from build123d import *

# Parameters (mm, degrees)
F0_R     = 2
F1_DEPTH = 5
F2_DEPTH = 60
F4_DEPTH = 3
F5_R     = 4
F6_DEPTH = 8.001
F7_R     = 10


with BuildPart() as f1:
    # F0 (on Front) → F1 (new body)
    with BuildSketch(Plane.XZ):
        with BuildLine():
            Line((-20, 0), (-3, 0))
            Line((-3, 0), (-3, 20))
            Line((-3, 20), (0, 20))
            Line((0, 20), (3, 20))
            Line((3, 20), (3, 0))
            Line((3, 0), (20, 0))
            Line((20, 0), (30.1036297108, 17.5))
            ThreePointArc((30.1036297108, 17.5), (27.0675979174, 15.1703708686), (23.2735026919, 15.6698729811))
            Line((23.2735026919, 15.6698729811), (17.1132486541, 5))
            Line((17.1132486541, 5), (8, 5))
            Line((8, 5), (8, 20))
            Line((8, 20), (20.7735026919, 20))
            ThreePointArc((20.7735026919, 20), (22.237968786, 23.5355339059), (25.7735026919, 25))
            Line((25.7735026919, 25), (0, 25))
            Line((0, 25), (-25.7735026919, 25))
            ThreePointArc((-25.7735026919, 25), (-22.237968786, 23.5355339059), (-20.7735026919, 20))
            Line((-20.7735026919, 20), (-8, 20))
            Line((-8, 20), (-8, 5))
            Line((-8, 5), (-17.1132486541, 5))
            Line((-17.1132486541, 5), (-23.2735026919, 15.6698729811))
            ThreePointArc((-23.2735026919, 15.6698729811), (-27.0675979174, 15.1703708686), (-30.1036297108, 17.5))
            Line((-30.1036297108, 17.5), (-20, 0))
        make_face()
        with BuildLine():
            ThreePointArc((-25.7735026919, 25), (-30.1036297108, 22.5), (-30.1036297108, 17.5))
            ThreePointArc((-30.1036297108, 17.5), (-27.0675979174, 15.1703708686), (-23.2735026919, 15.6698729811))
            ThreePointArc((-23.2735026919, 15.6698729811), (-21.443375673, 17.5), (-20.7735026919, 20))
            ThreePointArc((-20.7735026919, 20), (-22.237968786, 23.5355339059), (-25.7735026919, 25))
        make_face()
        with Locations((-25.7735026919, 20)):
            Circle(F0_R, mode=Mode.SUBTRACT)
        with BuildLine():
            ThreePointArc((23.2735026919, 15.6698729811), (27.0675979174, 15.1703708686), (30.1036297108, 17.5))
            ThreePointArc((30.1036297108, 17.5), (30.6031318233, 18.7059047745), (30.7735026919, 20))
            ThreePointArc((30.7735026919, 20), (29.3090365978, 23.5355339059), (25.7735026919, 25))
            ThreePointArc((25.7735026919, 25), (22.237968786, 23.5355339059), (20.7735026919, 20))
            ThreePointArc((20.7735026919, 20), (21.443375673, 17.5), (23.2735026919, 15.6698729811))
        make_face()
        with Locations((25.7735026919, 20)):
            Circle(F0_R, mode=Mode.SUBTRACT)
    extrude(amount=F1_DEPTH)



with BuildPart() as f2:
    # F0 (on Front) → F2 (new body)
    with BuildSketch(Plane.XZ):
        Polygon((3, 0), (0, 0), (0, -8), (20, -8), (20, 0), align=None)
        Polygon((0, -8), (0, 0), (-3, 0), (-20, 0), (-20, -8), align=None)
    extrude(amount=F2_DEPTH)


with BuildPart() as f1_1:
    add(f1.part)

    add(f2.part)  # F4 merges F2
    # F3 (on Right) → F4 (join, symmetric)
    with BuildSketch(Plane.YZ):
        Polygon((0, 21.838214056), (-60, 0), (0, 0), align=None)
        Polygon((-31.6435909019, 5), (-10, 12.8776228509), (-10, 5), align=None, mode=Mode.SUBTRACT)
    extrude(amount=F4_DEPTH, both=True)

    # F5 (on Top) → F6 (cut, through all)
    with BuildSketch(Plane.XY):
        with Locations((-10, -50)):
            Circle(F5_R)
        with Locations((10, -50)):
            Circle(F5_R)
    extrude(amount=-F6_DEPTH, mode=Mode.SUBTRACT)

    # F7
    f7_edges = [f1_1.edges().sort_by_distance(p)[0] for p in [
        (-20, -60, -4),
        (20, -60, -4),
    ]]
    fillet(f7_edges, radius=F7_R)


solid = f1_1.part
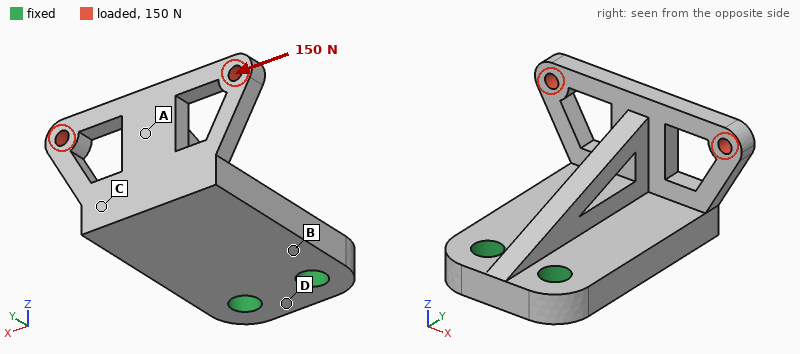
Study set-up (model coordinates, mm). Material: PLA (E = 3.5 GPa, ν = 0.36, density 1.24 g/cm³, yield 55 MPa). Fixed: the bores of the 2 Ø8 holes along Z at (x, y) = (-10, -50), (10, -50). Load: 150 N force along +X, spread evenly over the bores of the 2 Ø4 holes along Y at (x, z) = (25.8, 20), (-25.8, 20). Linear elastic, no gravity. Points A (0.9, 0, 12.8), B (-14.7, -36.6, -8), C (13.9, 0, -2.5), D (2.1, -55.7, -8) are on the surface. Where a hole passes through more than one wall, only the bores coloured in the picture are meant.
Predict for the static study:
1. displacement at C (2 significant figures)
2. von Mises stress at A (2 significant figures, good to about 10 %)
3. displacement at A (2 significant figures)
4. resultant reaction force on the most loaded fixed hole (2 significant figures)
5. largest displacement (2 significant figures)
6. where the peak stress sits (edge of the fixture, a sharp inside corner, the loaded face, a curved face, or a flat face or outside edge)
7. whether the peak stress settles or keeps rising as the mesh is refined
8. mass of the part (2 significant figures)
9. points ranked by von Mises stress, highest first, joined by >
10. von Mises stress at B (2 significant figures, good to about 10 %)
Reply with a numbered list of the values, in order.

1. 0.20 mm
2. 4.0 MPa
3. 0.30 mm
4. 320 N
5. 0.65 mm
6. edge of the fixture
7. keeps rising
8. 32 g
9. B > A > C > D
10. 5.5 MPa
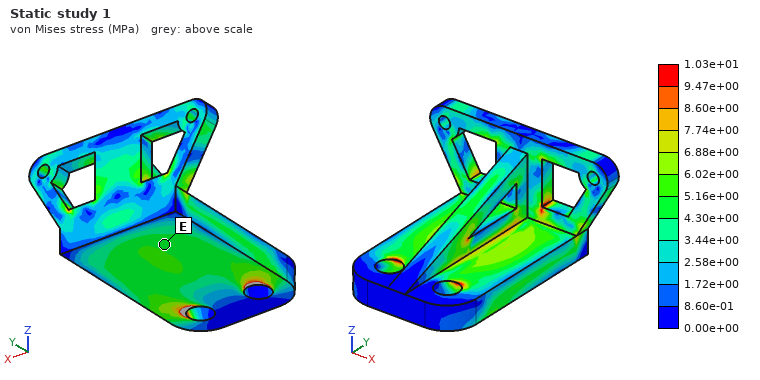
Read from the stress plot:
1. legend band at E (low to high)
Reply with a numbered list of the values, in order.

1. 4.30e+00 to 5.16e+00 MPa
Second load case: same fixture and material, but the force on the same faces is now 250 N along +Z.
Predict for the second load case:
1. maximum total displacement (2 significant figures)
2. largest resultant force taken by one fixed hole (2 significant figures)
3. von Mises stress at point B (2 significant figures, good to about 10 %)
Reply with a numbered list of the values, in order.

1. 1.1 mm
2. 130 N
3. 12 MPa
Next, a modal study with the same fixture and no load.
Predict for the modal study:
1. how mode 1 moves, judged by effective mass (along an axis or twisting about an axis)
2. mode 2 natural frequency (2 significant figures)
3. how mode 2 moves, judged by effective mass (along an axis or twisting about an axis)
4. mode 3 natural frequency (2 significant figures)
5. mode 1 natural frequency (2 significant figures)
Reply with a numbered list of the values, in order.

1. along Z
2. 1100 Hz
3. along X
4. 1800 Hz
5. 750 Hz
